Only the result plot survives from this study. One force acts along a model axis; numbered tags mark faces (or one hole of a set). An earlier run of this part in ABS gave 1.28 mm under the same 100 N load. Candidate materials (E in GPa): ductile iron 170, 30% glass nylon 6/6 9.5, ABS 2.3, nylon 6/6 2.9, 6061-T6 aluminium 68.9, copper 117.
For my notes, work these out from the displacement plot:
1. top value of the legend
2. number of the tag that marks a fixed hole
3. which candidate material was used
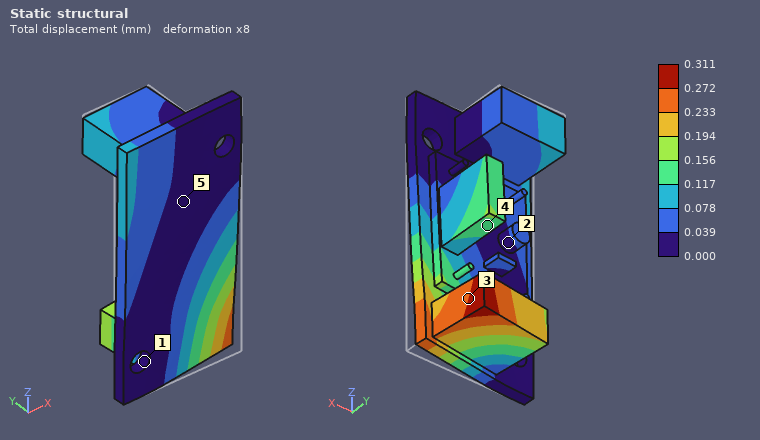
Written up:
0.311 mm
1
30% glass nylon 6/6
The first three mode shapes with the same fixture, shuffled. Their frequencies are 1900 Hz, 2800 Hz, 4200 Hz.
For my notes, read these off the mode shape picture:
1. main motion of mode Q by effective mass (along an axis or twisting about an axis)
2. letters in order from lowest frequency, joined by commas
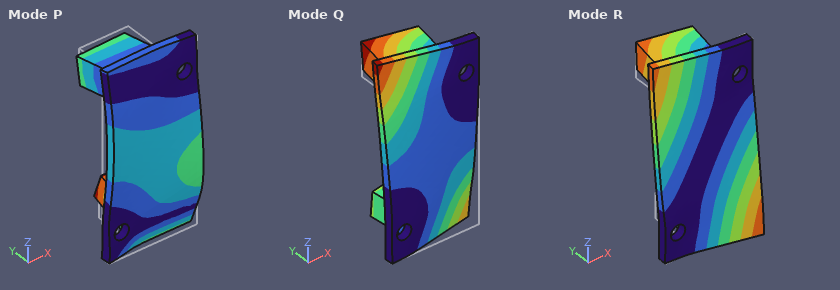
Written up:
along Y
R, Q, P
